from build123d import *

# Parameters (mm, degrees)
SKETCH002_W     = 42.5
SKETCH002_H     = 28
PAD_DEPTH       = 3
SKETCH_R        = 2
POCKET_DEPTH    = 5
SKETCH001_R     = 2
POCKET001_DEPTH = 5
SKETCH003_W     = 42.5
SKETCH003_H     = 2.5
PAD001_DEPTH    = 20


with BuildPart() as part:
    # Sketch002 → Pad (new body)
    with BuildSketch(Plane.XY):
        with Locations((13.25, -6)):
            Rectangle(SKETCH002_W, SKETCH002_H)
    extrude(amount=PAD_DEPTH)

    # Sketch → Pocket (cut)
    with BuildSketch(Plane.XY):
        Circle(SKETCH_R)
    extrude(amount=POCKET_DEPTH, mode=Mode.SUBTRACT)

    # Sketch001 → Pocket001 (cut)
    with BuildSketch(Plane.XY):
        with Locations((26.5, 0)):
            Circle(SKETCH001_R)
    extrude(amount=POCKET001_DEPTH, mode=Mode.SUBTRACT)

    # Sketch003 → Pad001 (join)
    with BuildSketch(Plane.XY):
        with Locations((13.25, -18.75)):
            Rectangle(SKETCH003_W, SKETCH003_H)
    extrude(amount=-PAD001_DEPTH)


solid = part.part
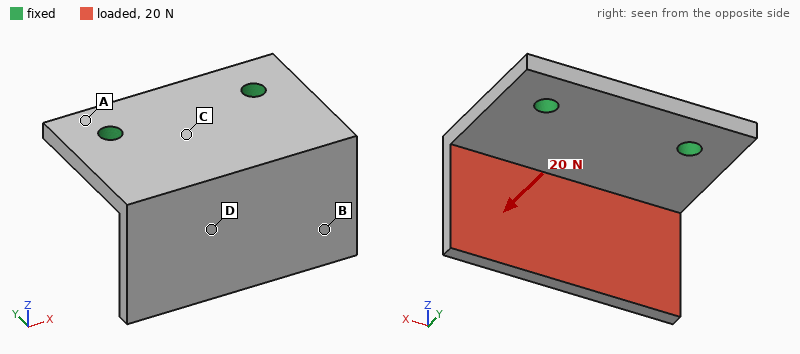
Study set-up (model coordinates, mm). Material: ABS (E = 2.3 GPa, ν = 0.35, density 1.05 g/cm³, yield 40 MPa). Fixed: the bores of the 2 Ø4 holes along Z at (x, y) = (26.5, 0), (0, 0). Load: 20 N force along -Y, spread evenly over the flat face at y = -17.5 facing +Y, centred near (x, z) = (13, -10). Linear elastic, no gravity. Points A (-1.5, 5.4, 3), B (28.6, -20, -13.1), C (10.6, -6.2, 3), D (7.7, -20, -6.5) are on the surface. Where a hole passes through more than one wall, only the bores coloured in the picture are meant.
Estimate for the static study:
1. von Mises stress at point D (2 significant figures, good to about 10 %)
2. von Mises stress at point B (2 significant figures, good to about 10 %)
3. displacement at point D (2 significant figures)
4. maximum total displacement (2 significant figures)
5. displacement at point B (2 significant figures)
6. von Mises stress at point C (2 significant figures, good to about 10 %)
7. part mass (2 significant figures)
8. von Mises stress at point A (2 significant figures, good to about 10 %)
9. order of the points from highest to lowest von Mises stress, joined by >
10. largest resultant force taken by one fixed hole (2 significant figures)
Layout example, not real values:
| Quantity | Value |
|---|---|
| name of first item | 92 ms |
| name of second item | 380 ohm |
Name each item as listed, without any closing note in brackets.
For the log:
| Quantity | Value |
|---|---|
| von Mises stress at point D | 1.8 MPa |
| von Mises stress at point B | 0.53 MPa |
| displacement at point D | 0.27 mm |
| maximum total displacement | 0.59 mm |
| displacement at point B | 0.42 mm |
| von Mises stress at point C | 2.6 MPa |
| part mass | 5.9 g |
| von Mises stress at point A | 0.92 MPa |
| order of the points from highest to lowest von Mises stress, joined by > | C > D > A > B |
| largest resultant force taken by one fixed hole | 10 N |
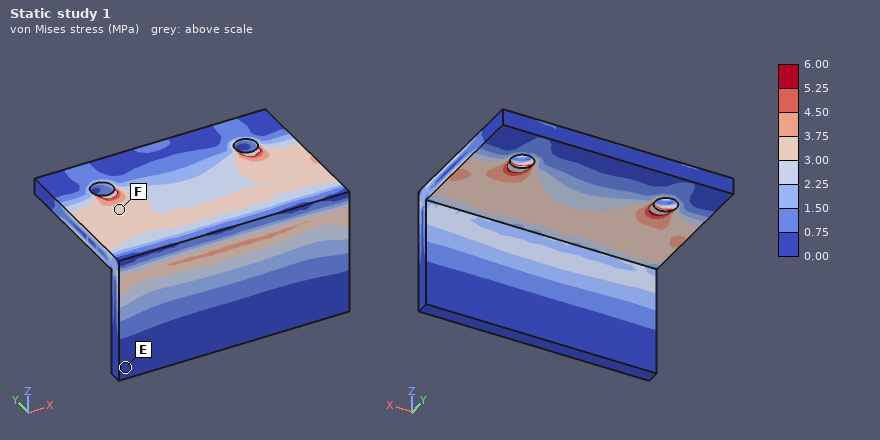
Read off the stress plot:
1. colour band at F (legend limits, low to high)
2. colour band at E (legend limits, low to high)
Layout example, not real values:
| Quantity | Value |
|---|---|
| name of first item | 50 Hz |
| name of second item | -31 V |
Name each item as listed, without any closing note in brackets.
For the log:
| Quantity | Value |
|---|---|
| colour band at F | 3.00 to 3.75 MPa |
| colour band at E | 0.00 to 0.75 MPa |
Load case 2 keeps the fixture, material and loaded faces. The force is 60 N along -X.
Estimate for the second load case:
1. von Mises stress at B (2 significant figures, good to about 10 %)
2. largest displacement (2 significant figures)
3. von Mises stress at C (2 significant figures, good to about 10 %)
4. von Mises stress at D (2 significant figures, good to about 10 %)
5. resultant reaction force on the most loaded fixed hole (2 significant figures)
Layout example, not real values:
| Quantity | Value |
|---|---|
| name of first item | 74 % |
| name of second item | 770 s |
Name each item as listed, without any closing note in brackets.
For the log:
| Quantity | Value |
|---|---|
| von Mises stress at B | 1.4 MPa |
| largest displacement | 0.57 mm |
| von Mises stress at C | 2.4 MPa |
| von Mises stress at D | 1.6 MPa |
| resultant reaction force on the most loaded fixed hole | 52 N |
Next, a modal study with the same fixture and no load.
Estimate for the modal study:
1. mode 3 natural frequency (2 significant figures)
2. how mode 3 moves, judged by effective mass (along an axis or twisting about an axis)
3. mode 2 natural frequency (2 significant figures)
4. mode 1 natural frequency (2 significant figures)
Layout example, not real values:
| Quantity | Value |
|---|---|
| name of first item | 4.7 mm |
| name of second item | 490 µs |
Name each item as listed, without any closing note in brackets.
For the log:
| Quantity | Value |
|---|---|
| mode 3 natural frequency | 1600 Hz |
| how mode 3 moves, judged by effective mass | along Z |
| mode 2 natural frequency | 1100 Hz |
| mode 1 natural frequency | 640 Hz |
